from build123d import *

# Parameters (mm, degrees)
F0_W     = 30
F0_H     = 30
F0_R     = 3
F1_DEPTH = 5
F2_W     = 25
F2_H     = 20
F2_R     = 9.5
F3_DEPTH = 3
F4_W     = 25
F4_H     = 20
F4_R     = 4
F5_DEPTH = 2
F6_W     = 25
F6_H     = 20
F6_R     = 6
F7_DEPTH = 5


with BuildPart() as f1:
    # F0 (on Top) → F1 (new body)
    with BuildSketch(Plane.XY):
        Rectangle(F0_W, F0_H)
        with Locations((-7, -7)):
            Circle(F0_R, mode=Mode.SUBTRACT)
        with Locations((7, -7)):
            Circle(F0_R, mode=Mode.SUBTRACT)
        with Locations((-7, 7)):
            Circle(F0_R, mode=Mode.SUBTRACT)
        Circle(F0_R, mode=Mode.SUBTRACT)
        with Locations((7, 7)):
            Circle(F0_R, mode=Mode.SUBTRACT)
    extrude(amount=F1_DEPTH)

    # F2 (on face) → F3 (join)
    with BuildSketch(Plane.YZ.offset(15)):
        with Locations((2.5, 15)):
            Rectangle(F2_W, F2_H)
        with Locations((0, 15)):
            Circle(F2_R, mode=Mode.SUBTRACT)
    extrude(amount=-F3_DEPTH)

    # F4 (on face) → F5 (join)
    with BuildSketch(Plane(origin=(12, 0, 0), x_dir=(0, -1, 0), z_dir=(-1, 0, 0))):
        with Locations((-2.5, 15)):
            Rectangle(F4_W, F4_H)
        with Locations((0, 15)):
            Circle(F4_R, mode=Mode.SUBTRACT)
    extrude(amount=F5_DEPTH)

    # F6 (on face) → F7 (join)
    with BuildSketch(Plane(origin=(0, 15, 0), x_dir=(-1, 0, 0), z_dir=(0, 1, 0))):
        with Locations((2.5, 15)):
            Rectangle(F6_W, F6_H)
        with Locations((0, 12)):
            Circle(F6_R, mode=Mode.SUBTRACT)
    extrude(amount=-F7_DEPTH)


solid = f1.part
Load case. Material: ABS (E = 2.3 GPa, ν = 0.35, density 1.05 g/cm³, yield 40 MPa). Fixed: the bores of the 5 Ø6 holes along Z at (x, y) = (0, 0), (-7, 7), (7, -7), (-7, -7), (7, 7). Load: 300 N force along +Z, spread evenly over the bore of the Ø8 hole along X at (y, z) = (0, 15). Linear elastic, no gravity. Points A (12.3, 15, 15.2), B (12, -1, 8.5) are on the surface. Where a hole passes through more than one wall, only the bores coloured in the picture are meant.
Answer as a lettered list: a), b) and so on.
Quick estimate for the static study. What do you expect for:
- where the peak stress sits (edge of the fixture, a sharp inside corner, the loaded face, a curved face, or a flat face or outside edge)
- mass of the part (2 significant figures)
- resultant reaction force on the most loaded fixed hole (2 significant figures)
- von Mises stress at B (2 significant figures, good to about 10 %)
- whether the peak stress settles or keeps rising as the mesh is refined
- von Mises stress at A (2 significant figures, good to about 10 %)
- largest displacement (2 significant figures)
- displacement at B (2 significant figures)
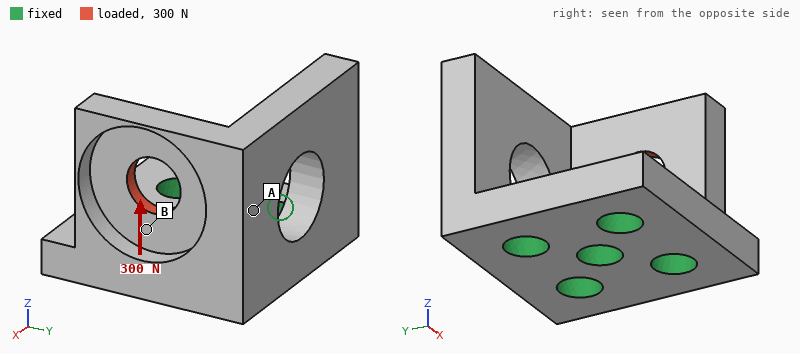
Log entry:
a) edge of the fixture
b) 7.6 g
c) 160 N
d) 5.5 MPa
e) keeps rising
f) 1.6 MPa
g) 79 µm
h) 21 µm
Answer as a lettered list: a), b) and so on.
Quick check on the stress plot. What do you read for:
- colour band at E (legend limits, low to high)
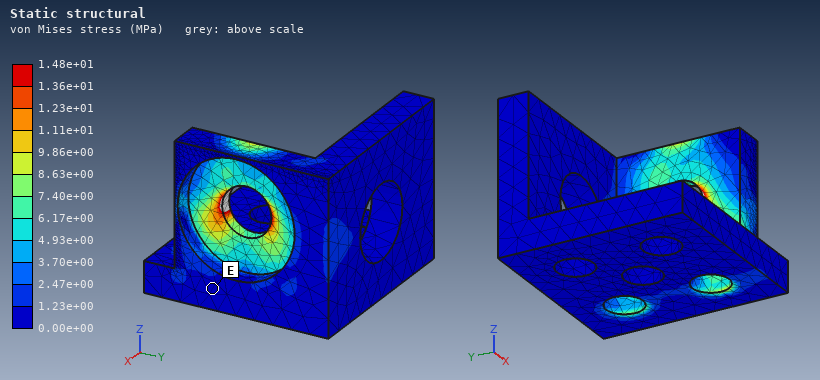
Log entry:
a) 0.00e+00 to 1.23e+00 MPa
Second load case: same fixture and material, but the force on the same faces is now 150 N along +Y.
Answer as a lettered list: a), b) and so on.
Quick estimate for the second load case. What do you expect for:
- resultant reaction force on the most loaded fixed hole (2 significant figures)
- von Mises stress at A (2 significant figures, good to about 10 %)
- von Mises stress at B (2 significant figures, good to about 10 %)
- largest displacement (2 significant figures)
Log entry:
a) 120 N
b) 0.94 MPa
c) 8.4 MPa
d) 0.11 mm
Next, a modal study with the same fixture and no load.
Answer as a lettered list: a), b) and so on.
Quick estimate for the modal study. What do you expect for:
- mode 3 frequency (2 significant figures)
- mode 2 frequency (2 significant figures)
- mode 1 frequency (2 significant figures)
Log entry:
a) 4200 Hz
b) 2900 Hz
c) 2500 Hz
